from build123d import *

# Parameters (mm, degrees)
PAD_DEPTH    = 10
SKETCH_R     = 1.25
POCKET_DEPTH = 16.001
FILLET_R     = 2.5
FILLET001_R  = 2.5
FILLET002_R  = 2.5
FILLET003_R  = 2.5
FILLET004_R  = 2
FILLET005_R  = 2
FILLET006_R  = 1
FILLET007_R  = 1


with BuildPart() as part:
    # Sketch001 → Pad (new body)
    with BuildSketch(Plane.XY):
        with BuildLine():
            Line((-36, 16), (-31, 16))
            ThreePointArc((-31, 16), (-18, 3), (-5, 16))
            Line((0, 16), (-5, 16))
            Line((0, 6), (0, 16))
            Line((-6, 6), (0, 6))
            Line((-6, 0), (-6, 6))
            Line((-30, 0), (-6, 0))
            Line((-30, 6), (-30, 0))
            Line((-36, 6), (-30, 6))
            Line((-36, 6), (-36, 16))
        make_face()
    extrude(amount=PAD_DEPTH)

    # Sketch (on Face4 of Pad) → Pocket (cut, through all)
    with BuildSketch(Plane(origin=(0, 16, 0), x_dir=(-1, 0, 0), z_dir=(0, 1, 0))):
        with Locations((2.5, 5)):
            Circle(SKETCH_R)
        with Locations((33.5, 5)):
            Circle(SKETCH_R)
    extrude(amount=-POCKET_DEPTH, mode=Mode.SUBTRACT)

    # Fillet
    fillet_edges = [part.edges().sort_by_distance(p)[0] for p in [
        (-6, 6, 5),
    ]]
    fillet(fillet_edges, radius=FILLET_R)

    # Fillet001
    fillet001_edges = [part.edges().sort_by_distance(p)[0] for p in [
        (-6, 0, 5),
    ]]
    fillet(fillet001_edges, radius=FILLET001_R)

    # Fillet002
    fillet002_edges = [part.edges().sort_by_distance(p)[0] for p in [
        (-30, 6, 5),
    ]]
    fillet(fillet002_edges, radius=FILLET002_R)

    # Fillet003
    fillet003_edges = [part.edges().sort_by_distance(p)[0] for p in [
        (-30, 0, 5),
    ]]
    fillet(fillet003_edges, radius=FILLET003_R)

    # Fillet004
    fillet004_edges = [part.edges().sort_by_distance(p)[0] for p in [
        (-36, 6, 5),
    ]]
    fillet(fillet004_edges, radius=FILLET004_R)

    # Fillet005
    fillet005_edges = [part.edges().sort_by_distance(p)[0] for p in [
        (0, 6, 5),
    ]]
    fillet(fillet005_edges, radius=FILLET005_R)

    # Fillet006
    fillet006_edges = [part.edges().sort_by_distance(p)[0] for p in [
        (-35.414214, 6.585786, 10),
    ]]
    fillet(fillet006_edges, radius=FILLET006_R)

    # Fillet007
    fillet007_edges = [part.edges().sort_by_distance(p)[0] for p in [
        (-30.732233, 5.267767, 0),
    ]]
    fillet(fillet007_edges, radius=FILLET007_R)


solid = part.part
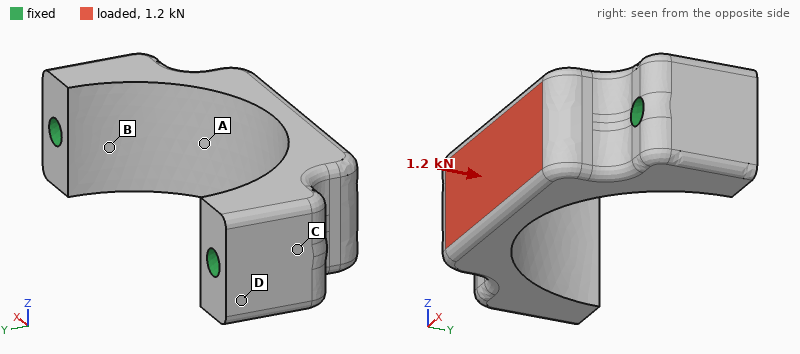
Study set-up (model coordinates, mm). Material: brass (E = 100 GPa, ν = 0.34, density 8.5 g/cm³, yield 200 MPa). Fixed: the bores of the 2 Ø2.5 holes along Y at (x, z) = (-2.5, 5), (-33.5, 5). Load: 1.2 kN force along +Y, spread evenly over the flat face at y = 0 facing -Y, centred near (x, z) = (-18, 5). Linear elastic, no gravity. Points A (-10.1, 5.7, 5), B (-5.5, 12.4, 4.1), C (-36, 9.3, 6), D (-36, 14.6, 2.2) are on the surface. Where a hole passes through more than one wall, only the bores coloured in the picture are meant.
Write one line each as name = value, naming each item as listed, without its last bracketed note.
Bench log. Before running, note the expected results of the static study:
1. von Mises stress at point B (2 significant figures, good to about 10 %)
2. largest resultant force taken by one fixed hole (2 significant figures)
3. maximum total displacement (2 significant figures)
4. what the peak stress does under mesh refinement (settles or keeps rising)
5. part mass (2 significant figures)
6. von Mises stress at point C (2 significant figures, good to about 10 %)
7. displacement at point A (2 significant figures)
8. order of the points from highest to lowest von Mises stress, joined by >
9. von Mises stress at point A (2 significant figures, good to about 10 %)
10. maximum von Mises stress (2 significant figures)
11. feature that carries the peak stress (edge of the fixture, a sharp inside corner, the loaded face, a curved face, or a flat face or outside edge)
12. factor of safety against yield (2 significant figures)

von Mises stress at point B = 16 MPa
largest resultant force taken by one fixed hole = 880 N
maximum total displacement = 9.0 µm
what the peak stress does under mesh refinement = settles
part mass = 19 g
von Mises stress at point C = 9.2 MPa
displacement at point A = 3.5 µm
order of the points from highest to lowest von Mises stress, joined by > = A > B > C > D
von Mises stress at point A = 43 MPa
maximum von Mises stress = 55 MPa
feature that carries the peak stress = the loaded face
factor of safety against yield = 3.7
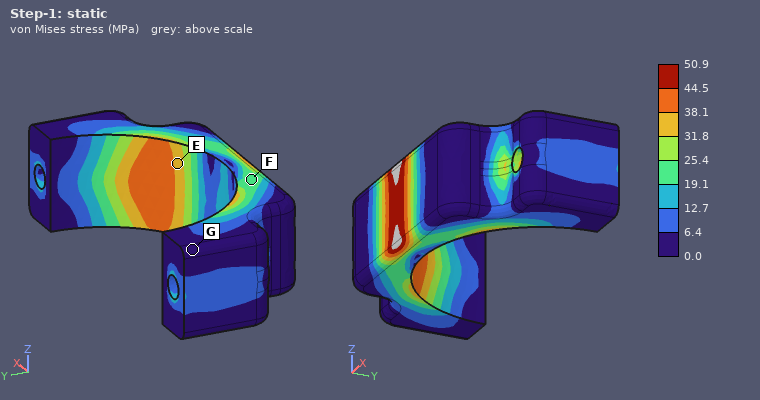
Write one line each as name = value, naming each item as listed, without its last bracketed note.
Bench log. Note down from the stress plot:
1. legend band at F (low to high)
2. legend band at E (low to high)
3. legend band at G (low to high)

legend band at F = 19.1 to 25.4 MPa
legend band at E = 31.8 to 38.1 MPa
legend band at G = 0.0 to 6.4 MPa
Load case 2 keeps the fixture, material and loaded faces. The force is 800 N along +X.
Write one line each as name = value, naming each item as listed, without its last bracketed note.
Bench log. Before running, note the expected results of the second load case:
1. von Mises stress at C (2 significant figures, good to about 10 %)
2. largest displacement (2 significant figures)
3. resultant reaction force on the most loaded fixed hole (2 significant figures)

von Mises stress at C = 6.5 MPa
largest displacement = 3.8 µm
resultant reaction force on the most loaded fixed hole = 450 N
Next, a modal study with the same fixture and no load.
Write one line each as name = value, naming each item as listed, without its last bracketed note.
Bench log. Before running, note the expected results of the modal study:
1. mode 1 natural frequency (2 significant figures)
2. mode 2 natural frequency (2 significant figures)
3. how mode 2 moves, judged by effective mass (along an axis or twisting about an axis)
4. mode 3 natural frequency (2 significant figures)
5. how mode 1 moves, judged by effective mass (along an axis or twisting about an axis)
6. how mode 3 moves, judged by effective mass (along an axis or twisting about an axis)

mode 1 natural frequency = 15 kHz
mode 2 natural frequency = 24 kHz
how mode 2 moves, judged by effective mass = along X
mode 3 natural frequency = 27 kHz
how mode 1 moves, judged by effective mass = along Z
how mode 3 moves, judged by effective mass = along Y
